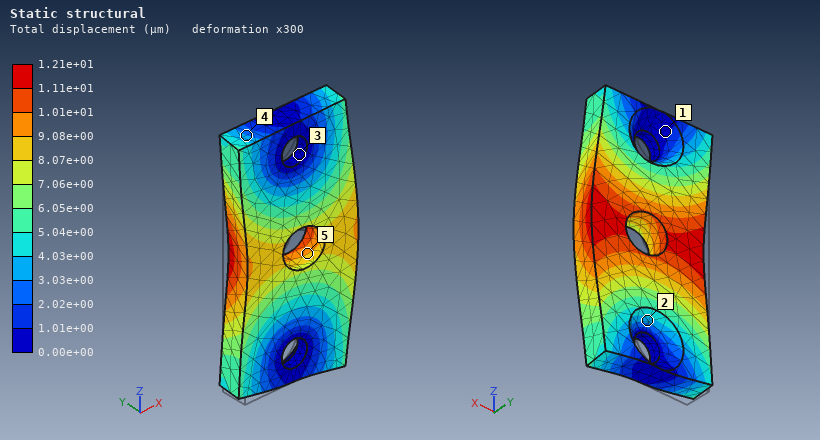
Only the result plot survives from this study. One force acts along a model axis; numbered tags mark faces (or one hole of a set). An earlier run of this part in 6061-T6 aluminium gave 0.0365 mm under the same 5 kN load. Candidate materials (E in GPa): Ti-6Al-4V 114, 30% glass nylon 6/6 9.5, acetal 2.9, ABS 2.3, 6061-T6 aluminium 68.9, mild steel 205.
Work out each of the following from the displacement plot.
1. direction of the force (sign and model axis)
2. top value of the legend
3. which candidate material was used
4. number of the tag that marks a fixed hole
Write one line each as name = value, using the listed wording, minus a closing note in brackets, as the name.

direction of the force = +X
top value of the legend = 1.21e+01 µm
which candidate material was used = mild steel
number of the tag that marks a fixed hole = 3
